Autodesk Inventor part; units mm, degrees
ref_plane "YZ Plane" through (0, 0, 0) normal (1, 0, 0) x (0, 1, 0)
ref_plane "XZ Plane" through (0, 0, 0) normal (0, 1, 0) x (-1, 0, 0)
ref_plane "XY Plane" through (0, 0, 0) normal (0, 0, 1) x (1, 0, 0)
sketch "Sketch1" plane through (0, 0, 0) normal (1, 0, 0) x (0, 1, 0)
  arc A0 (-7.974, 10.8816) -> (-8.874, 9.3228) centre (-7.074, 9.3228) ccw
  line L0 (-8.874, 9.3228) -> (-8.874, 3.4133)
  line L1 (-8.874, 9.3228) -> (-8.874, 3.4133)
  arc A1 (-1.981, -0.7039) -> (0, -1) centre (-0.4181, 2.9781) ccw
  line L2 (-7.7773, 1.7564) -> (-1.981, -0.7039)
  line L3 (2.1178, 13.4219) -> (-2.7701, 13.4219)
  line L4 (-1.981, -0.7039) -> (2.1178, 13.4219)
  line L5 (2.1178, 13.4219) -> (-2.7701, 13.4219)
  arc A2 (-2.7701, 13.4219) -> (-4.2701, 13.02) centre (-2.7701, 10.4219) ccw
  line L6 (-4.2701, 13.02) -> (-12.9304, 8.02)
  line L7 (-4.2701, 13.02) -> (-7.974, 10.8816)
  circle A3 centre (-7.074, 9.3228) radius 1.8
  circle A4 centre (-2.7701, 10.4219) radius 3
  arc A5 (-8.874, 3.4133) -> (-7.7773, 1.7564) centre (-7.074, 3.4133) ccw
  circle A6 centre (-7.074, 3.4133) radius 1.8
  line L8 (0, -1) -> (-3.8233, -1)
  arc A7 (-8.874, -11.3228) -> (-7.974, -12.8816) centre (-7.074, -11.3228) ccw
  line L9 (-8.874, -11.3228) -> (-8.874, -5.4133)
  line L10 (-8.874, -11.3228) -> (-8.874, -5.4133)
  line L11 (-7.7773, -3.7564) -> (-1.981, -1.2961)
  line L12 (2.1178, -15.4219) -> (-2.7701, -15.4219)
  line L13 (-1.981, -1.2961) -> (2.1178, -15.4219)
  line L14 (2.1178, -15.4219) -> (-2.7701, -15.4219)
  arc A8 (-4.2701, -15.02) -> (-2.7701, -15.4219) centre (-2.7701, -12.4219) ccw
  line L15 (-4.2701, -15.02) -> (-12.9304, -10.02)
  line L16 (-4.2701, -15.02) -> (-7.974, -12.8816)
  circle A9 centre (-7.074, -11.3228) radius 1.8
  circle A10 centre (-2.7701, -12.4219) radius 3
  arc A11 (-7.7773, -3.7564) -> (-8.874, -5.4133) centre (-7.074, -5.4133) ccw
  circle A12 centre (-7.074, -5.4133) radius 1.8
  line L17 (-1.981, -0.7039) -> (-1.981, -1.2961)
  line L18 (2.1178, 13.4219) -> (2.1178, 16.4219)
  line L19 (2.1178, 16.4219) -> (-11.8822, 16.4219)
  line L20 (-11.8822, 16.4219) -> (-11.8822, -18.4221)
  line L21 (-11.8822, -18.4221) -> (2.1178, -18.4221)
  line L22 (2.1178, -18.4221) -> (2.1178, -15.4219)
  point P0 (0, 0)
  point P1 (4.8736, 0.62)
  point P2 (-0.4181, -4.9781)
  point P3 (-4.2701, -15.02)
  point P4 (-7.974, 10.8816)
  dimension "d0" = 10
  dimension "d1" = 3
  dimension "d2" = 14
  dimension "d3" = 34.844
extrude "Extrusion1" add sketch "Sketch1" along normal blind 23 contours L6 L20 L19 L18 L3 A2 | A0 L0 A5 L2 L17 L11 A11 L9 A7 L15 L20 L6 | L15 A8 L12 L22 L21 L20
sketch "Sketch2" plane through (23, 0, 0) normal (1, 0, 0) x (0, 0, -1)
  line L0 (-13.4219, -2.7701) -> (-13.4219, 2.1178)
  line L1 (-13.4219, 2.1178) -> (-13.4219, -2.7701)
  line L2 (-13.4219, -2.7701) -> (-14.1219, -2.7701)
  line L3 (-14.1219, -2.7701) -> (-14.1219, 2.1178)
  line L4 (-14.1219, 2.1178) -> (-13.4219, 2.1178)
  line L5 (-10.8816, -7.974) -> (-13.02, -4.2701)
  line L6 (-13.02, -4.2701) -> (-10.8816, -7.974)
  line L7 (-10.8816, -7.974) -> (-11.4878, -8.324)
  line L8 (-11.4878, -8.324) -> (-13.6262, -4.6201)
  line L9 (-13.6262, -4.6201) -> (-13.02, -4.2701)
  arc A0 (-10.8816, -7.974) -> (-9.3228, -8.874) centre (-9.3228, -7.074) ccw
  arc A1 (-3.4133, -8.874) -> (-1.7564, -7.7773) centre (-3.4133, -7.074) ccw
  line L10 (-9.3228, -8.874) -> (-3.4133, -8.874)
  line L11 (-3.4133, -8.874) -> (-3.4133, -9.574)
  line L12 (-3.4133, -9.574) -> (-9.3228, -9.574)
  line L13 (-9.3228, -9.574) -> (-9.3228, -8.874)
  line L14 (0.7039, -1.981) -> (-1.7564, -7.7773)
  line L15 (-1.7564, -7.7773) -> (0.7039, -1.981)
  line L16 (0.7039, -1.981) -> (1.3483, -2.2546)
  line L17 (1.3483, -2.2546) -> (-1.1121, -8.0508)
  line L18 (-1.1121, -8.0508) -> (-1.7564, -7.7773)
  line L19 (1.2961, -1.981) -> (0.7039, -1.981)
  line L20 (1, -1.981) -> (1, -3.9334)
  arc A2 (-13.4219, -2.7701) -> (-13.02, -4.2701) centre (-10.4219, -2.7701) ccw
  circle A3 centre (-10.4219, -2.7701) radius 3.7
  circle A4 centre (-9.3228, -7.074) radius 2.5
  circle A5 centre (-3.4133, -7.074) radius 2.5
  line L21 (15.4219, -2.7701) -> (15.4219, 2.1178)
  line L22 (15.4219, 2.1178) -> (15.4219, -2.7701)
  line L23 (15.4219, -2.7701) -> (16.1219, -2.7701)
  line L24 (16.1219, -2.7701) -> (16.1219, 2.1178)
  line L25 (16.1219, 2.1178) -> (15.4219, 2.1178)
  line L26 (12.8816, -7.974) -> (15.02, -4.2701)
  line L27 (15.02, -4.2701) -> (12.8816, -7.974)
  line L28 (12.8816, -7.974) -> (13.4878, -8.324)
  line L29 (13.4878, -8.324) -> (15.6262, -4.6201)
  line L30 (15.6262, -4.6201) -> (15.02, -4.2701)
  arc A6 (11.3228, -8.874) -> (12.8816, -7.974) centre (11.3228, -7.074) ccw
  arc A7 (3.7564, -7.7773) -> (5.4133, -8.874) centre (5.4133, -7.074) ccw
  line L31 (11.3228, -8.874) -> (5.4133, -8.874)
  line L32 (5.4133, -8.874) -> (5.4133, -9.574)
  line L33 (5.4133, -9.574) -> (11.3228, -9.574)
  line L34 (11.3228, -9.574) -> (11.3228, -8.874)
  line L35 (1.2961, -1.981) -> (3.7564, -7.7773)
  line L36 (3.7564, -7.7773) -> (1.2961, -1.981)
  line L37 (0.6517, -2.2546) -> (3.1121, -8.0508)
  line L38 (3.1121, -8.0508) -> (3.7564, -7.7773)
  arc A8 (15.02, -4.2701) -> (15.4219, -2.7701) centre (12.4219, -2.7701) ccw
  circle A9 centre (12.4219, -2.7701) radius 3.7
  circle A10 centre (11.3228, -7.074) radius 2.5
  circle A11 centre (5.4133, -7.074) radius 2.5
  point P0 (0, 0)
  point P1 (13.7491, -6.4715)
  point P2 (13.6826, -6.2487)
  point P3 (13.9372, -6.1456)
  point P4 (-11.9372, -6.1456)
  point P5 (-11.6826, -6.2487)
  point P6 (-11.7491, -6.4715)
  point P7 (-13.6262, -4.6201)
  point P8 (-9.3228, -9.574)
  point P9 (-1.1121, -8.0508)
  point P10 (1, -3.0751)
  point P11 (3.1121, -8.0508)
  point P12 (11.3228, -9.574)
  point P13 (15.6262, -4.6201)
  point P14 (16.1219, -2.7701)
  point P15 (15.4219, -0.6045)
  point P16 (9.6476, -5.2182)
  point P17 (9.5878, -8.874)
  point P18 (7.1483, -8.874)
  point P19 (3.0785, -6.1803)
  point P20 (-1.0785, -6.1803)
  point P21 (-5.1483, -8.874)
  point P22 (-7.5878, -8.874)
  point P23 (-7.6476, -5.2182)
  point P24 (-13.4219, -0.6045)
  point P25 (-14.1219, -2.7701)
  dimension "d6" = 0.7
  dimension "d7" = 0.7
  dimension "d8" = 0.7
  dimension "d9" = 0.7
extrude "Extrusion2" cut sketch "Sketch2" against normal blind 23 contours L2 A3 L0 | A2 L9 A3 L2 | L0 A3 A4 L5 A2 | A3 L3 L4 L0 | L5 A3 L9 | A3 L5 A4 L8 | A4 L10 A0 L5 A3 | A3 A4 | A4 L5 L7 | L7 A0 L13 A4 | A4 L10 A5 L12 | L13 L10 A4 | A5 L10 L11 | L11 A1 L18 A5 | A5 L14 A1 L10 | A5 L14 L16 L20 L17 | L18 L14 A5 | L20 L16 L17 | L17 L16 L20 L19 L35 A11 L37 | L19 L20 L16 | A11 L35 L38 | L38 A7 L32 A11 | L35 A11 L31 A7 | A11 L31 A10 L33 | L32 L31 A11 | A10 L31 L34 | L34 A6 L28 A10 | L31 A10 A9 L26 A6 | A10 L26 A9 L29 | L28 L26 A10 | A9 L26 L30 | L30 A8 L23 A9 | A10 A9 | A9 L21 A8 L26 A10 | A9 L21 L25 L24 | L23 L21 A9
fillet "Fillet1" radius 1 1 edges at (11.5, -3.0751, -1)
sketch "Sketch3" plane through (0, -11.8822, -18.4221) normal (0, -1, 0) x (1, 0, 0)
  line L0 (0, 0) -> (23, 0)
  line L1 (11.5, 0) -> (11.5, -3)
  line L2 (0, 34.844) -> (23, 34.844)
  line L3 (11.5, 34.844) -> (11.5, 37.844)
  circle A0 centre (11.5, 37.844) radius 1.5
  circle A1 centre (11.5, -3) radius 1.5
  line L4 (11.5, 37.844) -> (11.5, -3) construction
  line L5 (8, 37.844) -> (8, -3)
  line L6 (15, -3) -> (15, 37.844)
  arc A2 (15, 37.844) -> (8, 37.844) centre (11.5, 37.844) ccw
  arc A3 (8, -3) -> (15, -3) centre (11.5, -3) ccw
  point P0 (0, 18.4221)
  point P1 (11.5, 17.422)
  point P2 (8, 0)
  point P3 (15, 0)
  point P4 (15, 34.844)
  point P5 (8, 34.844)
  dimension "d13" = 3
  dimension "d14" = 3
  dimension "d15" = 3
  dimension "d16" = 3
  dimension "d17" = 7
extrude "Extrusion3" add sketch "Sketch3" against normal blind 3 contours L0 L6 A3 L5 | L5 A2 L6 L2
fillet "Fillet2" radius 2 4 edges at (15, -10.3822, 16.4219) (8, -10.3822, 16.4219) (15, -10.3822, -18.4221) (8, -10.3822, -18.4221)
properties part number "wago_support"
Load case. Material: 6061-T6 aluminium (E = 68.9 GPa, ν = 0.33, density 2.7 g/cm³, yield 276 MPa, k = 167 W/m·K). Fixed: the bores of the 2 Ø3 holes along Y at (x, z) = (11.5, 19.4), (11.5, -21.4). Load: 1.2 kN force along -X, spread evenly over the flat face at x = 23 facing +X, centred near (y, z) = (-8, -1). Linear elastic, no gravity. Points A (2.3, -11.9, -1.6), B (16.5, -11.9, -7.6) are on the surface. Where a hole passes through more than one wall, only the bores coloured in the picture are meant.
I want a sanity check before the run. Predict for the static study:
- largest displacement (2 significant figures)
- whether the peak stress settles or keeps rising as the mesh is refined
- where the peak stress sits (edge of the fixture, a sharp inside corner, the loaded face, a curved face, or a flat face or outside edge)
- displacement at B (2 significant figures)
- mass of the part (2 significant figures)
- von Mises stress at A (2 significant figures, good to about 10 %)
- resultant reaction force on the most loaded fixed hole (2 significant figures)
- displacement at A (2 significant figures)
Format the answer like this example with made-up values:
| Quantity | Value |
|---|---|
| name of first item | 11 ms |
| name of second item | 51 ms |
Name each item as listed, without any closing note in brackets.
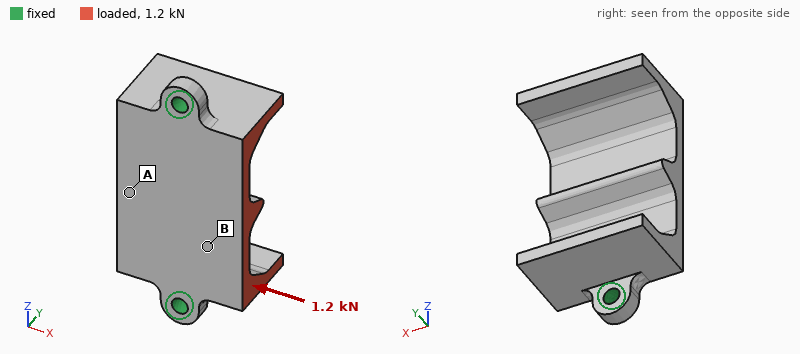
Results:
| Quantity | Value |
|---|---|
| largest displacement | 51 µm |
| whether the peak stress settles or keeps rising as the mesh is refined | keeps rising |
| where the peak stress sits | edge of the fixture |
| displacement at B | 14 µm |
| mass of the part | 11 g |
| von Mises stress at A | 22 MPa |
| resultant reaction force on the most loaded fixed hole | 600 N |
| displacement at A | 28 µm |
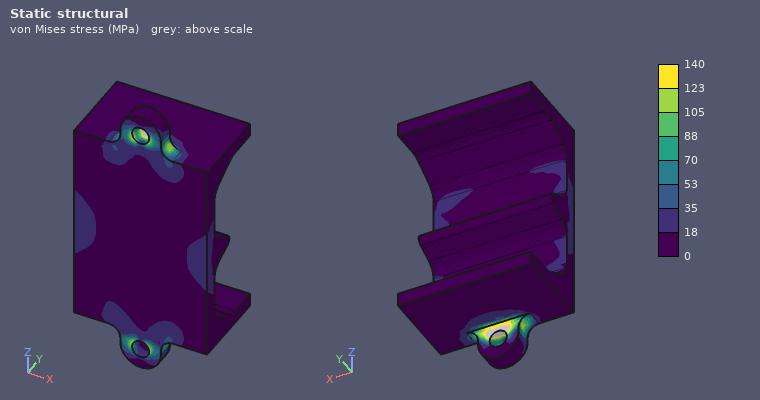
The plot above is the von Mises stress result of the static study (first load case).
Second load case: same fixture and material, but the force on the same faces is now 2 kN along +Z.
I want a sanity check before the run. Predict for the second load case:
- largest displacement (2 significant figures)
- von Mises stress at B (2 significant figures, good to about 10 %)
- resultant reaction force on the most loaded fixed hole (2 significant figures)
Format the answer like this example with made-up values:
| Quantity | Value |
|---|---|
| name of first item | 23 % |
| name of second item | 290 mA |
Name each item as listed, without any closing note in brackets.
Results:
| Quantity | Value |
|---|---|
| largest displacement | 86 µm |
| von Mises stress at B | 49 MPa |
| resultant reaction force on the most loaded fixed hole | 1.2 kN |
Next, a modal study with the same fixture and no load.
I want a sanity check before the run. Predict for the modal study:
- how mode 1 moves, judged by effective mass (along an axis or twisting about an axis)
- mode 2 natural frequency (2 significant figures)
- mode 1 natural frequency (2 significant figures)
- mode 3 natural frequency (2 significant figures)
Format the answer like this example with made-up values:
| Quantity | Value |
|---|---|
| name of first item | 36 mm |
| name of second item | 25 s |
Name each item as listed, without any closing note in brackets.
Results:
| Quantity | Value |
|---|---|
| how mode 1 moves, judged by effective mass | along Y |
| mode 2 natural frequency | 6100 Hz |
| mode 1 natural frequency | 5800 Hz |
| mode 3 natural frequency | 10 kHz |
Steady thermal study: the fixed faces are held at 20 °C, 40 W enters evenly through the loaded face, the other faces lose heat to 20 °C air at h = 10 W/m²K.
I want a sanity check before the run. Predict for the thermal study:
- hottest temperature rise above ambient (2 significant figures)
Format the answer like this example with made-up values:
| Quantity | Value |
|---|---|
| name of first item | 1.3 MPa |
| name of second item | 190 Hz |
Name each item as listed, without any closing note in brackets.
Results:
| Quantity | Value |
|---|---|
| hottest temperature rise above ambient | 42 K |
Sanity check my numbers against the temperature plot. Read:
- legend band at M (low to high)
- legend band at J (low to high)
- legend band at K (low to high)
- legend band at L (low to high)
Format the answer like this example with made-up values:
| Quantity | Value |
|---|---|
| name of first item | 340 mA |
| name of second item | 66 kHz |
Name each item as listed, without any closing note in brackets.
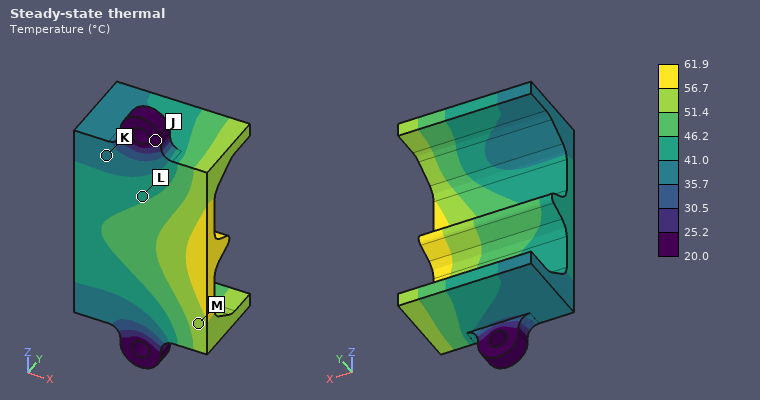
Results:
| Quantity | Value |
|---|---|
| legend band at M | 51.4 to 56.7 °C |
| legend band at J | 20.0 to 25.2 °C |
| legend band at K | 35.7 to 41.0 °C |
| legend band at L | 41.0 to 46.2 °C |
